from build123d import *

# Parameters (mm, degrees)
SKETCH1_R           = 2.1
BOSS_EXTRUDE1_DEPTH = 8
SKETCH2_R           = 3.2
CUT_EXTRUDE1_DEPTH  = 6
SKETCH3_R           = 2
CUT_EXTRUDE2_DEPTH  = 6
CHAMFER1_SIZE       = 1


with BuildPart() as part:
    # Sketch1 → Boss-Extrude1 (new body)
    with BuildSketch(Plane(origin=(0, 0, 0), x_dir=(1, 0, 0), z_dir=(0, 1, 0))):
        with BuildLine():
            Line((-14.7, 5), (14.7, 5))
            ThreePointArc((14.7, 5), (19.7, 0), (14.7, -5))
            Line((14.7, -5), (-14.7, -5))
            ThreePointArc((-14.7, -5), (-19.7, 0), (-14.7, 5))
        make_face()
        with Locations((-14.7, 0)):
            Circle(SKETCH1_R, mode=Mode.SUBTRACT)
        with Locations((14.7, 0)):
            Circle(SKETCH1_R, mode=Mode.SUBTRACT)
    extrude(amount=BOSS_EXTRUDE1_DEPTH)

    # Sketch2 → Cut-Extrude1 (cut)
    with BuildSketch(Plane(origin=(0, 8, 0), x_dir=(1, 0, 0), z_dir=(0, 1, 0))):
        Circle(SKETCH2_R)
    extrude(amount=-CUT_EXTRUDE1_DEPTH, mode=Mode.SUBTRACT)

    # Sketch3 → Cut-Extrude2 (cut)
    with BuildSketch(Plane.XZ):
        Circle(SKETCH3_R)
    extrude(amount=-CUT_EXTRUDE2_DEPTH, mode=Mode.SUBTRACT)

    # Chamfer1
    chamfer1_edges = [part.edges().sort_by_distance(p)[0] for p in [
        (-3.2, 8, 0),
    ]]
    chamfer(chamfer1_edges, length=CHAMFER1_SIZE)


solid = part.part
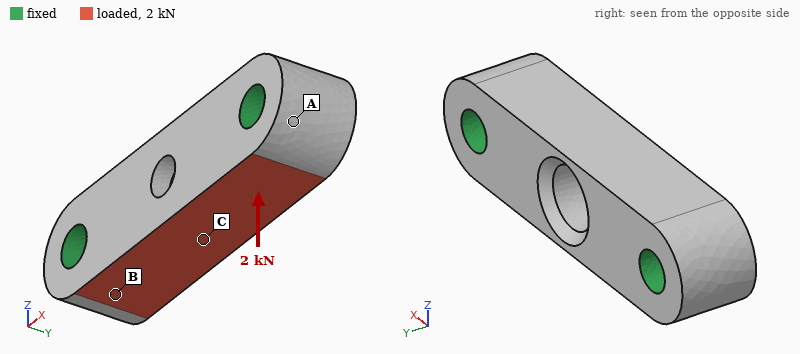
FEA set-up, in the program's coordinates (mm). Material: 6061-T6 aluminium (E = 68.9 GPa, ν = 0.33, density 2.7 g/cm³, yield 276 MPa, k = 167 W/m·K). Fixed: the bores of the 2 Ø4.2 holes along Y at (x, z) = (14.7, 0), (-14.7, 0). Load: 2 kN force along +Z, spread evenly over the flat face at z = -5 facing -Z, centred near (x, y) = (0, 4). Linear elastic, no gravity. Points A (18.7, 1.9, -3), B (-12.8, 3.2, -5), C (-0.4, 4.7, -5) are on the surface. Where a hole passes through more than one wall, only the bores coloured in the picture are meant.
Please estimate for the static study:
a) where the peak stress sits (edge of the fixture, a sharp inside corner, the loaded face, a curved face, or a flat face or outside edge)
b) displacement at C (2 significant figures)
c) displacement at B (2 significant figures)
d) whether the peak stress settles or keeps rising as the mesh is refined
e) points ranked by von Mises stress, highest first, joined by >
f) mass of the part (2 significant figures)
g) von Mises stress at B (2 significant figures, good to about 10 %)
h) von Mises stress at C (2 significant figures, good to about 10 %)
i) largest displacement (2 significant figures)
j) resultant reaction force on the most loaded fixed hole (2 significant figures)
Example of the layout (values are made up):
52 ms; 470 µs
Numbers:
edge of the fixture; 8.5 µm; 2.2 µm; keeps rising; C > B > A; 6.8 g; 20 MPa; 38 MPa; 9.5 µm; 1.0 kN
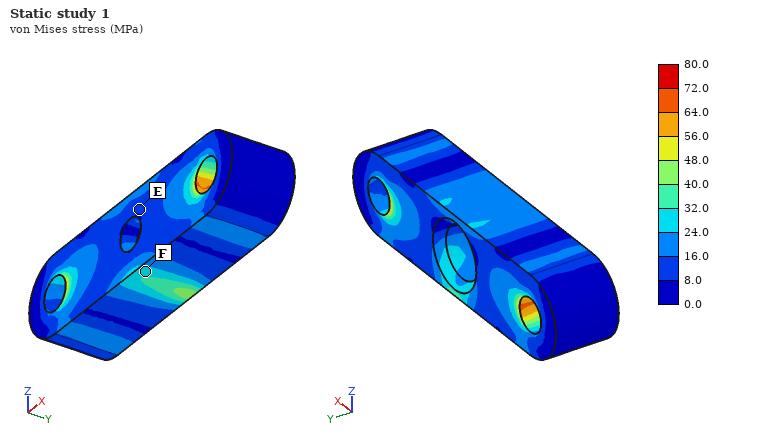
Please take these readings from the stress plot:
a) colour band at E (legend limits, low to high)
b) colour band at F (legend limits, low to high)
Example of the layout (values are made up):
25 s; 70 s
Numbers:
8.0 to 16.0 MPa; 24.0 to 32.0 MPa
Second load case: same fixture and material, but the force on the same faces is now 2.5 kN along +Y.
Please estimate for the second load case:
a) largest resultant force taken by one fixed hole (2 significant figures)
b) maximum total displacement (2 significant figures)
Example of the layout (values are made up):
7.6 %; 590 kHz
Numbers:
1.3 kN; 25 µm
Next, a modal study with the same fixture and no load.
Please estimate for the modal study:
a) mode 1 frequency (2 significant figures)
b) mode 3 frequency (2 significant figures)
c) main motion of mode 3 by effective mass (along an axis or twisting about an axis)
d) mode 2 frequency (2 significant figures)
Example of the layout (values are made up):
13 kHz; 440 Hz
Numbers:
40 kHz; 54 kHz; twisting about X; 41 kHz
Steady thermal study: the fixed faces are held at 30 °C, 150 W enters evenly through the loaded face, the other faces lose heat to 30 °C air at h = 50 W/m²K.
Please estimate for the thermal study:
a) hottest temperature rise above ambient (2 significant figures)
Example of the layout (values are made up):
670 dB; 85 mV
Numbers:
59 K
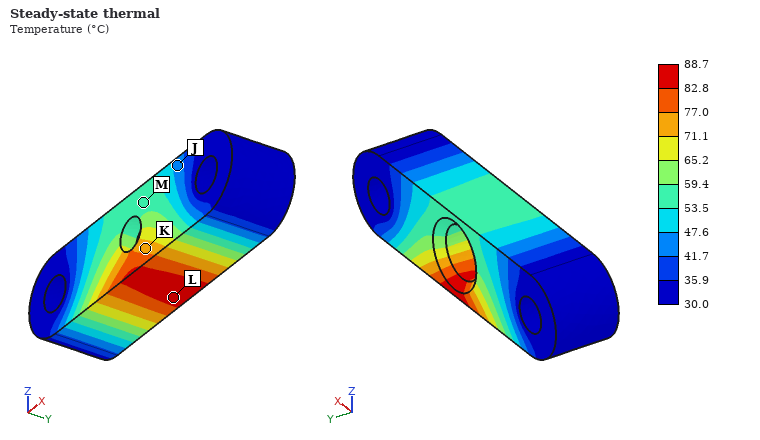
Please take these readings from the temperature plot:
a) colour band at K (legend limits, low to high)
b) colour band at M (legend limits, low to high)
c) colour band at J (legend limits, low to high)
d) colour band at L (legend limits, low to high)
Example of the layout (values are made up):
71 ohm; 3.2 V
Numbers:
71.1 to 77.0 °C; 53.5 to 59.4 °C; 41.7 to 47.6 °C; 82.8 to 88.7 °C
